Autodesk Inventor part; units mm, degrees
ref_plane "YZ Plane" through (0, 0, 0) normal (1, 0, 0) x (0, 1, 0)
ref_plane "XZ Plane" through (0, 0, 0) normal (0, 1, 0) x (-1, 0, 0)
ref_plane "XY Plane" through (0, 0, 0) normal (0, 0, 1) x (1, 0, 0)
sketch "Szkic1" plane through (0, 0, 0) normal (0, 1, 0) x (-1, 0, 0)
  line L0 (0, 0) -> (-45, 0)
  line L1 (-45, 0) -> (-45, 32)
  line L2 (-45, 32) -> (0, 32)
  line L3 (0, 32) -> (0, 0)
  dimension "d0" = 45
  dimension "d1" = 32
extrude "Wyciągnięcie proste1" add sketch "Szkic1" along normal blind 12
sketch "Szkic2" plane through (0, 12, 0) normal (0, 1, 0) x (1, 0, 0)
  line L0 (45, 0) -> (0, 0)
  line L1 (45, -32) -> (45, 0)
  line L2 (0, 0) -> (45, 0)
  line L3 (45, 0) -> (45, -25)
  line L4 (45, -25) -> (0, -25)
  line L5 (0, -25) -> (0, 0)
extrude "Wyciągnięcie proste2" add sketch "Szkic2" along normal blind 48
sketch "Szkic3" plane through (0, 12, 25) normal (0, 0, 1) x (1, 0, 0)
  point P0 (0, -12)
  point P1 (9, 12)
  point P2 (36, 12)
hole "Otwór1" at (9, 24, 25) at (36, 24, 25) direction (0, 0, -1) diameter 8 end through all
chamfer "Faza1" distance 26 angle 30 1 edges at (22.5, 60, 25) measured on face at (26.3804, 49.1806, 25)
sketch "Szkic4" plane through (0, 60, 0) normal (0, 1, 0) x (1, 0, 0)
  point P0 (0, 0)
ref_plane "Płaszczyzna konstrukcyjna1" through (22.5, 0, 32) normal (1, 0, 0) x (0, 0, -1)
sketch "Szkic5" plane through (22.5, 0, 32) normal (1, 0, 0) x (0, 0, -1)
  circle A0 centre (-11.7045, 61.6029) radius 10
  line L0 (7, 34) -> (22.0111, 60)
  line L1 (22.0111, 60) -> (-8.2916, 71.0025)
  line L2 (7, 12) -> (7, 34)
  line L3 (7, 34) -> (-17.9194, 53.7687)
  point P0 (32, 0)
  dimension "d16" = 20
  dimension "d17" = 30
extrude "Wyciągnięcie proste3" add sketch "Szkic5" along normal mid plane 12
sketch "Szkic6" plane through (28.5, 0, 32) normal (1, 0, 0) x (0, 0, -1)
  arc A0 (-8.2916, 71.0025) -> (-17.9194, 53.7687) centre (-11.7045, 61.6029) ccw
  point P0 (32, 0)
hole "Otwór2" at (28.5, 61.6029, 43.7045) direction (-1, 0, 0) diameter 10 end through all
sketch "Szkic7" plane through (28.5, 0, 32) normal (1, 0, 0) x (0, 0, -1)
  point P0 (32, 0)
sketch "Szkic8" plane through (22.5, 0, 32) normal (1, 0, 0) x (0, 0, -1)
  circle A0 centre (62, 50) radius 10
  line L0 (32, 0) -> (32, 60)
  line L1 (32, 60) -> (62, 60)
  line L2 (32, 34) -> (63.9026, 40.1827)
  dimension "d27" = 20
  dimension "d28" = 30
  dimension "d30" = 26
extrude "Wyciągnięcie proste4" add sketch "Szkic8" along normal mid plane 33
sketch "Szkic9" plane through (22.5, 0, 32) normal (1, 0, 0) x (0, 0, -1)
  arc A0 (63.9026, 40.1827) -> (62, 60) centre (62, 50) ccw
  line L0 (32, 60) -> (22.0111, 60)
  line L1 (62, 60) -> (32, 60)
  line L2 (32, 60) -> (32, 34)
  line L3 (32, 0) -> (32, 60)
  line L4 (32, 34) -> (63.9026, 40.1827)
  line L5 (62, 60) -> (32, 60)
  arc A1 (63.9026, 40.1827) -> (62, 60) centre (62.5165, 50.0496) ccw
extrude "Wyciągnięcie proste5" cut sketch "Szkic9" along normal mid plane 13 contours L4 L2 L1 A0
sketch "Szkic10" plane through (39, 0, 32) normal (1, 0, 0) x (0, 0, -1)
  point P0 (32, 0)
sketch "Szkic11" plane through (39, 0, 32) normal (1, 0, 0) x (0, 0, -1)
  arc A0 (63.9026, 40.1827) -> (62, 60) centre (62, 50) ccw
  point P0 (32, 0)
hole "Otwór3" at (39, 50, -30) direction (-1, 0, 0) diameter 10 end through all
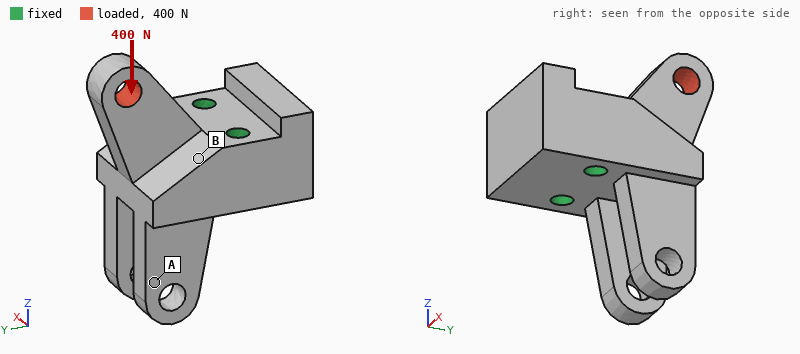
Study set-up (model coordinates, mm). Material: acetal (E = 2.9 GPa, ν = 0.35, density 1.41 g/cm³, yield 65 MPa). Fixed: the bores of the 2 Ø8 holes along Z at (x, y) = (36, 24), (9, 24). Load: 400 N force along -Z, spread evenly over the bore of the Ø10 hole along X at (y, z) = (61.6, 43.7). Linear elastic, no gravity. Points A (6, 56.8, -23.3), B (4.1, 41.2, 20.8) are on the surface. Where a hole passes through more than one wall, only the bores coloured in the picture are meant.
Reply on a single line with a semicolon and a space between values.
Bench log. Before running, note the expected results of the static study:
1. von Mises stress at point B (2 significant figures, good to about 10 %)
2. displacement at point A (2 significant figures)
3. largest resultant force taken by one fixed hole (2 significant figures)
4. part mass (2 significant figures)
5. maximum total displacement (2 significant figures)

1.8 MPa; 0.070 mm; 200 N; 120 g; 0.18 mm
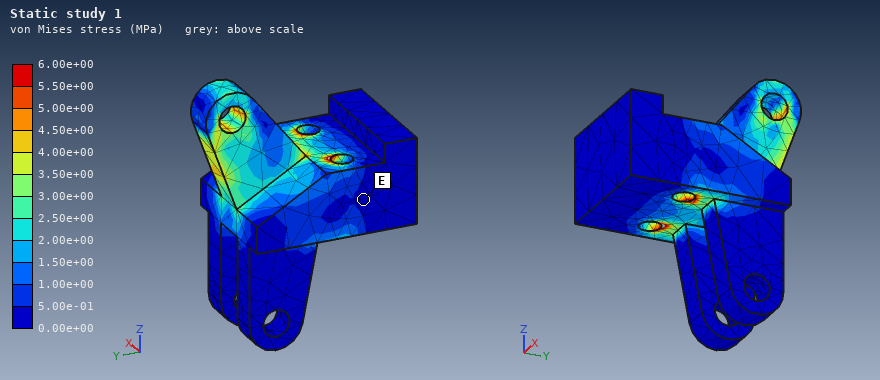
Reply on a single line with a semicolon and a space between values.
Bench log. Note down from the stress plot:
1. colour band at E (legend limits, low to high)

0.00e+00 to 5.00e-01 MPa
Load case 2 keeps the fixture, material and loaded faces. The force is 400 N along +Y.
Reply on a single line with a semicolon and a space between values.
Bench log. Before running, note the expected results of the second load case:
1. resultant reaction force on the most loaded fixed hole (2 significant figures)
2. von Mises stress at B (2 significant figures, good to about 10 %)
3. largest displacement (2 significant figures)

230 N; 1.7 MPa; 0.24 mm
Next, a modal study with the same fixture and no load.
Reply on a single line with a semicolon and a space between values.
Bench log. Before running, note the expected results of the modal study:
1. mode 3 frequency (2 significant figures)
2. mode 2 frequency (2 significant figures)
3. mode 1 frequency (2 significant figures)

1800 Hz; 1500 Hz; 1500 Hz
